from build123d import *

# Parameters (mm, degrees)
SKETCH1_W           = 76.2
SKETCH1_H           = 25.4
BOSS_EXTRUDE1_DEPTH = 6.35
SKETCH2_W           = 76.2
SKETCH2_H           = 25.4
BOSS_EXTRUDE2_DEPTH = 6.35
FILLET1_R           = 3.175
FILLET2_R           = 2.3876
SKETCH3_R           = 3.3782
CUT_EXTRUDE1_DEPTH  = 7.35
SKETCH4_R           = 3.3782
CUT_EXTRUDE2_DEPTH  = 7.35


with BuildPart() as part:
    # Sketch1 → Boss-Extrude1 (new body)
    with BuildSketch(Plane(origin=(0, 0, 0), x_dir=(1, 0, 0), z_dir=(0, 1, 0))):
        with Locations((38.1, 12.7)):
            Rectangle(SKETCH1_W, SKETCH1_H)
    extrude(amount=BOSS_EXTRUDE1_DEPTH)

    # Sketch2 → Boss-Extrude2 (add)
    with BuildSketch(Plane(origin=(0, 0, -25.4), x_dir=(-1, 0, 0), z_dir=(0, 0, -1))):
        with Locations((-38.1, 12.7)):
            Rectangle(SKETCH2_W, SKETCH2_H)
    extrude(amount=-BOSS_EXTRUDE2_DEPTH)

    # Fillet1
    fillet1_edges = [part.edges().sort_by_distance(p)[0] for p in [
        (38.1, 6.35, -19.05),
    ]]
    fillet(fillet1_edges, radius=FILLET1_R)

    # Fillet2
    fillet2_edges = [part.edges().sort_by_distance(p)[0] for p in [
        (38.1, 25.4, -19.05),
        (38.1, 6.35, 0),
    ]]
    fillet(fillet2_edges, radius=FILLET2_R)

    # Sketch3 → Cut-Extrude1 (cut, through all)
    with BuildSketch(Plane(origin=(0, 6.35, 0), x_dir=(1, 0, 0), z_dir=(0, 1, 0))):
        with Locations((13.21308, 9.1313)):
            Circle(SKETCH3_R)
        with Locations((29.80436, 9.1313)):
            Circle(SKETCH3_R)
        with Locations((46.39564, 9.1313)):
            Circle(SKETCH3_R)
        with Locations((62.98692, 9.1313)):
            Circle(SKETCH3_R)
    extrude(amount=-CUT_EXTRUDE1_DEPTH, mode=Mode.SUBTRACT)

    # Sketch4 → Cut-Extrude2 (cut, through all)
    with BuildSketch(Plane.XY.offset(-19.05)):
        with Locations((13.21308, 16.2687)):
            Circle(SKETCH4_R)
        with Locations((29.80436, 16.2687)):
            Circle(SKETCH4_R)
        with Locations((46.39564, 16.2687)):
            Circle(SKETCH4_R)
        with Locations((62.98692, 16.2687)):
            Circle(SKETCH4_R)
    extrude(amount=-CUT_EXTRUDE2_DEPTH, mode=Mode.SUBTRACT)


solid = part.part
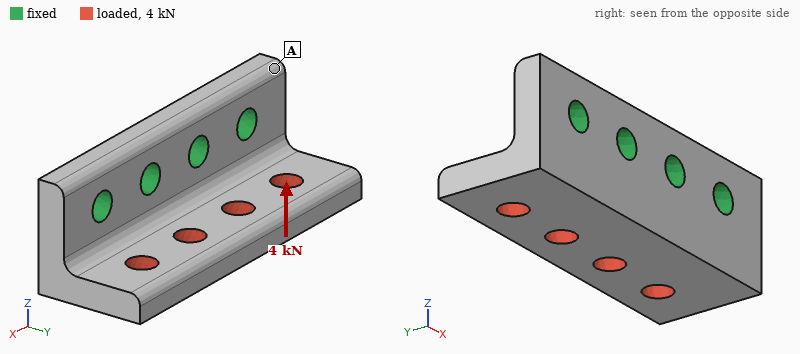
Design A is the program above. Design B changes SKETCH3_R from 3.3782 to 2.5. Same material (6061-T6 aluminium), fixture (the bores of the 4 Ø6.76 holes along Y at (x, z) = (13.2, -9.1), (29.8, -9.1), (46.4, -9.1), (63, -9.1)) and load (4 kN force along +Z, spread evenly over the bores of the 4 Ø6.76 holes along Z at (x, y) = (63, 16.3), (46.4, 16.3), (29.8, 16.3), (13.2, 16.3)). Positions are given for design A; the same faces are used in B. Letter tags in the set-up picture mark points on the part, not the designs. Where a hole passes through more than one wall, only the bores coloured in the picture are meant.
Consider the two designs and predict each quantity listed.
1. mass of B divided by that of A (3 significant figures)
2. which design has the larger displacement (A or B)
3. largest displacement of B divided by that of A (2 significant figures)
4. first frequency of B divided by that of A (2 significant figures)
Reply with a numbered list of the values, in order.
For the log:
1. 1.02
2. B
3. 1.1
4. 0.93
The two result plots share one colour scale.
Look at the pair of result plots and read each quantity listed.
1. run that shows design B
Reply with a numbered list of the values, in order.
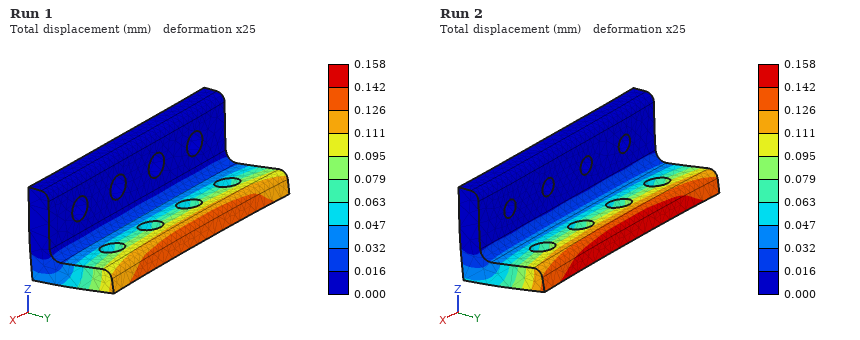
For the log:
1. Run 2
